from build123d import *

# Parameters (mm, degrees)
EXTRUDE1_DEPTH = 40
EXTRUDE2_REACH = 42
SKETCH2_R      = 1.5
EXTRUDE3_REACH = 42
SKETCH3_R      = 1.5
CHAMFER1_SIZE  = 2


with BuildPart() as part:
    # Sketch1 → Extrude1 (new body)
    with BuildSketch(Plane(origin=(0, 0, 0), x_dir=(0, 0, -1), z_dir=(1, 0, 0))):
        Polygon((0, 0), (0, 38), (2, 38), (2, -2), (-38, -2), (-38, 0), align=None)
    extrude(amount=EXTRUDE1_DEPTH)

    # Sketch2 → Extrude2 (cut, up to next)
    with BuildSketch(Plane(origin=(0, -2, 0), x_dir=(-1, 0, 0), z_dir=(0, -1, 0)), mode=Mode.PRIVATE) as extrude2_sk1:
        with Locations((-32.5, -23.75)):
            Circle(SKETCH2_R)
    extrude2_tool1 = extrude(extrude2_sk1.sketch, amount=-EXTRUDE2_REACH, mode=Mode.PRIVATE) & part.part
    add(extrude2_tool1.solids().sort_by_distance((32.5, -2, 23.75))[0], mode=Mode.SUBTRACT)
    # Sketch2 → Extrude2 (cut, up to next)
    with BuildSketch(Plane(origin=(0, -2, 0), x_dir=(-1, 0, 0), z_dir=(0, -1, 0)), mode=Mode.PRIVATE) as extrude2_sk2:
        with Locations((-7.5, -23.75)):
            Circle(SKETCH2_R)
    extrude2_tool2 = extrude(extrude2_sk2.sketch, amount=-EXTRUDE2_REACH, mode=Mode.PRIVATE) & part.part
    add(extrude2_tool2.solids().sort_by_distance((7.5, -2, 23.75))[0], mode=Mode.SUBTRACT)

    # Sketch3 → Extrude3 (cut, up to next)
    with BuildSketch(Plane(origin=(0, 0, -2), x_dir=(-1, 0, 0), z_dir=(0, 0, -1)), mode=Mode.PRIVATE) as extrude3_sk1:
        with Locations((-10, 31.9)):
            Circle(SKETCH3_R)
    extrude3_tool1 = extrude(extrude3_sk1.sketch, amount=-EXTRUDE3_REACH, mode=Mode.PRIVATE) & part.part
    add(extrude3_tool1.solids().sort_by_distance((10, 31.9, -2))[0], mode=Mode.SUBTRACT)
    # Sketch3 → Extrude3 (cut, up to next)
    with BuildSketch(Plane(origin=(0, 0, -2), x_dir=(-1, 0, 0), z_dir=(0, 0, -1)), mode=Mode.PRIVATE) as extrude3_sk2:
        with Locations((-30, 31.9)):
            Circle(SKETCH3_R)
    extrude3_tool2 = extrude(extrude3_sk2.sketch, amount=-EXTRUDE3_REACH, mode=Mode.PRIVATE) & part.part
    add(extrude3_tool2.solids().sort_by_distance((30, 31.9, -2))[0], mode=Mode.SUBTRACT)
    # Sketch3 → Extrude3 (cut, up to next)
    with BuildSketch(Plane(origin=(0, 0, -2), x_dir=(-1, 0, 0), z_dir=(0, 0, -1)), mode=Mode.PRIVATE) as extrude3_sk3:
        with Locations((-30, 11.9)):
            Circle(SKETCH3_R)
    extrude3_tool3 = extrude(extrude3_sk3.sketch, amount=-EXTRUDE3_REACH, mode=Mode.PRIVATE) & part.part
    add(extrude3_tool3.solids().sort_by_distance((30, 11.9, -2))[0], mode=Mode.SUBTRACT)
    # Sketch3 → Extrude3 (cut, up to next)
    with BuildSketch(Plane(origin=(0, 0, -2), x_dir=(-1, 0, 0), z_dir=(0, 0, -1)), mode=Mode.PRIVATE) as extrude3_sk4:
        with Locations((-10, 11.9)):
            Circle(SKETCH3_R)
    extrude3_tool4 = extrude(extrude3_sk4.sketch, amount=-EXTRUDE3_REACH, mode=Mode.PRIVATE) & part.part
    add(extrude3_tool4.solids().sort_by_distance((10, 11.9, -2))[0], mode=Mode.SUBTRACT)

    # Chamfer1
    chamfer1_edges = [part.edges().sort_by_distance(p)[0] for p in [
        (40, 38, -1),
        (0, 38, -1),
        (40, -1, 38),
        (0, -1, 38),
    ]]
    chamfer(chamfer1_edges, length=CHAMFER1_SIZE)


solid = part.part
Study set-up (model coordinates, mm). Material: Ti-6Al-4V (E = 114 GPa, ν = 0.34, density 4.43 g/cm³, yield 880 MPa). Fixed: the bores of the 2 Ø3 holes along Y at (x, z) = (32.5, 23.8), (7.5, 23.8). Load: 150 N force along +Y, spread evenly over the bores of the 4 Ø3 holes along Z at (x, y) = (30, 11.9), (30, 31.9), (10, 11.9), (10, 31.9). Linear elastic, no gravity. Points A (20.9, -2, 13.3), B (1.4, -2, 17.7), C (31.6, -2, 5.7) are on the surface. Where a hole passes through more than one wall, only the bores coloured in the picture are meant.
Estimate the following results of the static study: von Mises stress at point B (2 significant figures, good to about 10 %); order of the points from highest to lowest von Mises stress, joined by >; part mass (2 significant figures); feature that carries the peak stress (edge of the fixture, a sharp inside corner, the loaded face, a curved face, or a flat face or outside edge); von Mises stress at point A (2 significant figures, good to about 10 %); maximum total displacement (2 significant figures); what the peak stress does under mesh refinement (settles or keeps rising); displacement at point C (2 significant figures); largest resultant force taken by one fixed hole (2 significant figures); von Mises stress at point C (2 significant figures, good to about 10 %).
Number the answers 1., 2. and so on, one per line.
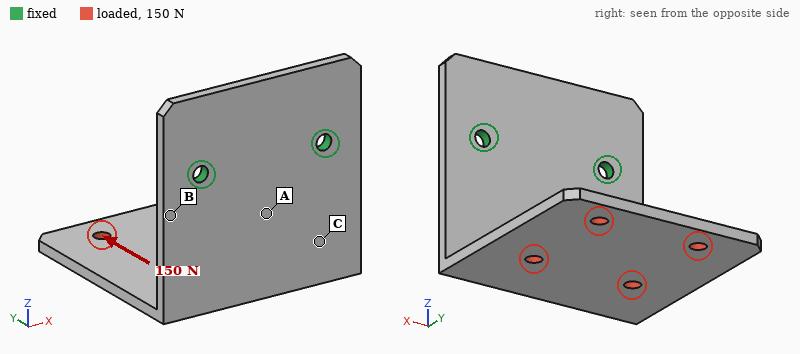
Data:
1. 110 MPa
2. B > A > C
3. 27 g
4. edge of the fixture
5. 69 MPa
6. 0.63 mm
7. keeps rising
8. 0.15 mm
9. 75 N
10. 35 MPa
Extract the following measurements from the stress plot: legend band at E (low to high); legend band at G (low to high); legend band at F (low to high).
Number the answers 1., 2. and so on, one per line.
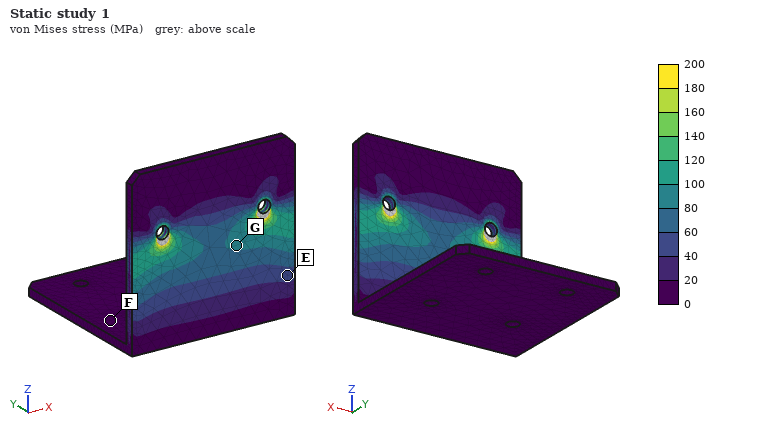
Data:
1. 40 to 60 MPa
2. 80 to 100 MPa
3. 0 to 20 MPa
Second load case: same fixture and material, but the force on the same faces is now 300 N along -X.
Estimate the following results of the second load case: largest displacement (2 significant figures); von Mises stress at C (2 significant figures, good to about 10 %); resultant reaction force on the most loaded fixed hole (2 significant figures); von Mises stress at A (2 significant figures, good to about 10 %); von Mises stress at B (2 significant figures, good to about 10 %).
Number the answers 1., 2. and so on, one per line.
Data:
1. 0.79 mm
2. 120 MPa
3. 400 N
4. 120 MPa
5. 160 MPa
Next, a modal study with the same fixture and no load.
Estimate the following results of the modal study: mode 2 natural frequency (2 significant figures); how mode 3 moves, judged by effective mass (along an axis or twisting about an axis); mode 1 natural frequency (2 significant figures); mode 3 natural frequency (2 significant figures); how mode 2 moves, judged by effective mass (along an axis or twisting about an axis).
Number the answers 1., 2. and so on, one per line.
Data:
1. 1000 Hz
2. along Y
3. 540 Hz
4. 1600 Hz
5. along X
